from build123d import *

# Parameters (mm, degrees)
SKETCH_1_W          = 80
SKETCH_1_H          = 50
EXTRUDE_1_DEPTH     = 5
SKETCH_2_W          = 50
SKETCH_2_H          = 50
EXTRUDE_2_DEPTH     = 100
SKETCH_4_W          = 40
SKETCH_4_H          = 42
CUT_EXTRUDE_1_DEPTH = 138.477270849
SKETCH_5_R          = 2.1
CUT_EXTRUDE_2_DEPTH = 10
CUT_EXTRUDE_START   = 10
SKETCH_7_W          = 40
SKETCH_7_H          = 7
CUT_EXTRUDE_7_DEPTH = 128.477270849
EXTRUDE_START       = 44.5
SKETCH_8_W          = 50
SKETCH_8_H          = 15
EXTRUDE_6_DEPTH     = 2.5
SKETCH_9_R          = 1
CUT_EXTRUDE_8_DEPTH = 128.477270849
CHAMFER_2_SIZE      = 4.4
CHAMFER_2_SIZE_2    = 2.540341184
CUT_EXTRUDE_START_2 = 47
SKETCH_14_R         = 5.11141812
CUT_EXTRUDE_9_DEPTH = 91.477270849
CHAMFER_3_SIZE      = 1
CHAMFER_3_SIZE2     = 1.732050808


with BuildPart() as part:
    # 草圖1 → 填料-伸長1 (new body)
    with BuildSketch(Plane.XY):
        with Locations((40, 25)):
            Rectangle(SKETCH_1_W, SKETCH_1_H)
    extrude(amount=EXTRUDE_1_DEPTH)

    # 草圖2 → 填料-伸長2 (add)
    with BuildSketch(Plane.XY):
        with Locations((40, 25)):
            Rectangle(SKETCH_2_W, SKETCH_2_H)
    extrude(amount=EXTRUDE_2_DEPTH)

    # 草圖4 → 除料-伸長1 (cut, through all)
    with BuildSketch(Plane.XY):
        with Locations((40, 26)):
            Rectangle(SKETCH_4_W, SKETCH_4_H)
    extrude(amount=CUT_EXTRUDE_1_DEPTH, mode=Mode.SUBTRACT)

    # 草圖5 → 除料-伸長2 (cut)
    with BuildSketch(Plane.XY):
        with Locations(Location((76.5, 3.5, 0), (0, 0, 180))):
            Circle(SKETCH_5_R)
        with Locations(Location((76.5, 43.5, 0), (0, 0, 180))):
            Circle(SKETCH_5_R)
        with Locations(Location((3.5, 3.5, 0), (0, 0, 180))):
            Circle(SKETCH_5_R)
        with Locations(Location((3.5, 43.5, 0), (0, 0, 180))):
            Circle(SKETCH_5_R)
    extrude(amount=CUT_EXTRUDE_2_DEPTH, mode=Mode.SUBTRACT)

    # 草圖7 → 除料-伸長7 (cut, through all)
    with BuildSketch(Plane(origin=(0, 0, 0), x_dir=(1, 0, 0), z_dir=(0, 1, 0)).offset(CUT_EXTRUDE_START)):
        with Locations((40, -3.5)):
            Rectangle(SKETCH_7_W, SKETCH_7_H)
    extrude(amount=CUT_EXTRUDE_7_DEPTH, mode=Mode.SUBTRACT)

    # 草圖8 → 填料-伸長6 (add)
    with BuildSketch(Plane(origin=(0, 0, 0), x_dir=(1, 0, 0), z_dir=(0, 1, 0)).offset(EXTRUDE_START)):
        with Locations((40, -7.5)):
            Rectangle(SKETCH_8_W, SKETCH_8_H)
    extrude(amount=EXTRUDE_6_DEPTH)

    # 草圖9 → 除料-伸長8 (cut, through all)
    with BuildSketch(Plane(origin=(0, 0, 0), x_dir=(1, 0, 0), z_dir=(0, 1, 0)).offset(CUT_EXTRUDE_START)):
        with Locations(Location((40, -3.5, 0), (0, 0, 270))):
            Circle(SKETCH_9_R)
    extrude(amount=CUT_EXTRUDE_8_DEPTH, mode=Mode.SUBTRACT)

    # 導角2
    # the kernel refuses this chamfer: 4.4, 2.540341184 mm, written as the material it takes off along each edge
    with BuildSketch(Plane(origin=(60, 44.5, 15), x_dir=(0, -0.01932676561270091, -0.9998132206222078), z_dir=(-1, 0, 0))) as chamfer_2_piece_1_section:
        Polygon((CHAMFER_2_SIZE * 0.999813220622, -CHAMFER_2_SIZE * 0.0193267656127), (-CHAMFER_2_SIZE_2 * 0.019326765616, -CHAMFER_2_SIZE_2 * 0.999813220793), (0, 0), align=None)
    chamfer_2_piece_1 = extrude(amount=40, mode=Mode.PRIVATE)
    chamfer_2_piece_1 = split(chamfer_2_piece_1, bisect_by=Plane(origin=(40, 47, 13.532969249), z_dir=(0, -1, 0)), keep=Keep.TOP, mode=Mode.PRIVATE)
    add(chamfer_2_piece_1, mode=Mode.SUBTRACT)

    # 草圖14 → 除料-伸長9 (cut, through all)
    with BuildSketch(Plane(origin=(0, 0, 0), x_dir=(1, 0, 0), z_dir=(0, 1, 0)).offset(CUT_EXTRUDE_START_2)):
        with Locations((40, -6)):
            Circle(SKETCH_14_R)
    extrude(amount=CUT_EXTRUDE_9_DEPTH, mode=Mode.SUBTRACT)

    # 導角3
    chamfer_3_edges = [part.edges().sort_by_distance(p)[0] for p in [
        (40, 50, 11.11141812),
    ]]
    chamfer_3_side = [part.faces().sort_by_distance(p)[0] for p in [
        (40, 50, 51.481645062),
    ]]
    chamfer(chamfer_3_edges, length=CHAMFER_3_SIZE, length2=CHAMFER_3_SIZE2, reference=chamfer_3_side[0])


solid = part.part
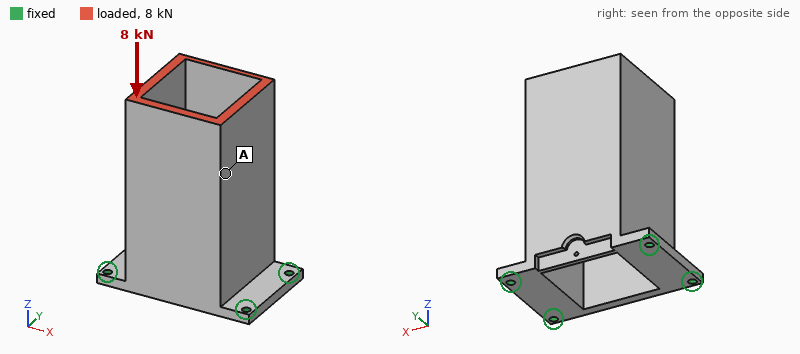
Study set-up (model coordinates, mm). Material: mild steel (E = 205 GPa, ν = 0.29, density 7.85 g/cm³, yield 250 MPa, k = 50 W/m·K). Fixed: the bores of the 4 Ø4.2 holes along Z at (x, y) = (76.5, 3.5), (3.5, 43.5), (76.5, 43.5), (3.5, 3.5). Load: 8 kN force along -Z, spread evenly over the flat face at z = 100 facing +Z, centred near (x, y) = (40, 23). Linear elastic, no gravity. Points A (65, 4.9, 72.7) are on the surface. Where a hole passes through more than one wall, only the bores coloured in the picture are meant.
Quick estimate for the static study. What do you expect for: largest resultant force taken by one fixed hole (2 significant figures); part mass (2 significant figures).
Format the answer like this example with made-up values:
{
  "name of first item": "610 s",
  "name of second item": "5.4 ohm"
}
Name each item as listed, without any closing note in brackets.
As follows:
{
  "largest resultant force taken by one fixed hole": "2.3 kN",
  "part mass": "700 g"
}
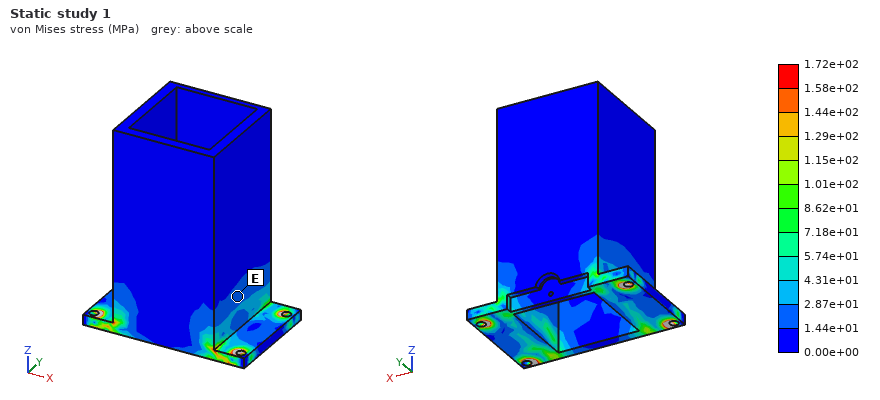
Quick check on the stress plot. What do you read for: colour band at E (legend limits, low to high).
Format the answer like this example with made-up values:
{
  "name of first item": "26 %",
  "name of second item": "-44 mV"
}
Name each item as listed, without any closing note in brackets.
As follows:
{
  "colour band at E": "1.44e+01 to 2.87e+01 MPa"
}
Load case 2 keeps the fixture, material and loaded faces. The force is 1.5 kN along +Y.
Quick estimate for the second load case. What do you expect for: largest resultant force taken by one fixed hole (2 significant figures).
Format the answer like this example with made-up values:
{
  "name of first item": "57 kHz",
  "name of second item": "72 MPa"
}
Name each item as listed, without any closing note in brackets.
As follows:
{
  "largest resultant force taken by one fixed hole": "2.2 kN"
}
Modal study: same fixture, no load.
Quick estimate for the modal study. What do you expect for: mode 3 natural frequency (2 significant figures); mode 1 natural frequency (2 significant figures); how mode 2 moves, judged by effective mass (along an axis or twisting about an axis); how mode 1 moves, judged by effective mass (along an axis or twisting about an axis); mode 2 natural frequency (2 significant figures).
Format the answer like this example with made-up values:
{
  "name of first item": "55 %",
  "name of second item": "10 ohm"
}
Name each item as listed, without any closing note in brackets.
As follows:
{
  "mode 3 natural frequency": "3400 Hz",
  "mode 1 natural frequency": "1200 Hz",
  "how mode 2 moves, judged by effective mass": "along X",
  "how mode 1 moves, judged by effective mass": "along Y",
  "mode 2 natural frequency": "1800 Hz"
}
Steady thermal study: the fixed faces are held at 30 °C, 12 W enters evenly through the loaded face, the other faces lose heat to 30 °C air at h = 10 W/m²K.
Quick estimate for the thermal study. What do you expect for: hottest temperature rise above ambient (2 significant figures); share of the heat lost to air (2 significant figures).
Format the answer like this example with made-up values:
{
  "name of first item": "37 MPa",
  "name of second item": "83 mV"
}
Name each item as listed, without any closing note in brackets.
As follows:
{
  "hottest temperature rise above ambient": "27 K",
  "share of the heat lost to air": "45 %"
}
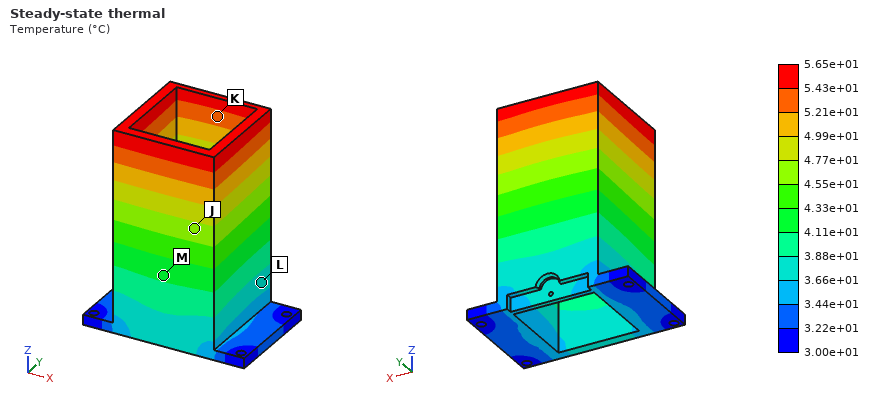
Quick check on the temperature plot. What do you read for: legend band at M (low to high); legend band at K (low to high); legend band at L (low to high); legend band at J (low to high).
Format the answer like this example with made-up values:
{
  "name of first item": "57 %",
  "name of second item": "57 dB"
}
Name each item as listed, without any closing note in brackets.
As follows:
{
  "legend band at M": "4.11e+01 to 4.33e+01 °C",
  "legend band at K": "5.21e+01 to 5.43e+01 °C",
  "legend band at L": "3.66e+01 to 3.88e+01 °C",
  "legend band at J": "4.55e+01 to 4.77e+01 °C"
}
